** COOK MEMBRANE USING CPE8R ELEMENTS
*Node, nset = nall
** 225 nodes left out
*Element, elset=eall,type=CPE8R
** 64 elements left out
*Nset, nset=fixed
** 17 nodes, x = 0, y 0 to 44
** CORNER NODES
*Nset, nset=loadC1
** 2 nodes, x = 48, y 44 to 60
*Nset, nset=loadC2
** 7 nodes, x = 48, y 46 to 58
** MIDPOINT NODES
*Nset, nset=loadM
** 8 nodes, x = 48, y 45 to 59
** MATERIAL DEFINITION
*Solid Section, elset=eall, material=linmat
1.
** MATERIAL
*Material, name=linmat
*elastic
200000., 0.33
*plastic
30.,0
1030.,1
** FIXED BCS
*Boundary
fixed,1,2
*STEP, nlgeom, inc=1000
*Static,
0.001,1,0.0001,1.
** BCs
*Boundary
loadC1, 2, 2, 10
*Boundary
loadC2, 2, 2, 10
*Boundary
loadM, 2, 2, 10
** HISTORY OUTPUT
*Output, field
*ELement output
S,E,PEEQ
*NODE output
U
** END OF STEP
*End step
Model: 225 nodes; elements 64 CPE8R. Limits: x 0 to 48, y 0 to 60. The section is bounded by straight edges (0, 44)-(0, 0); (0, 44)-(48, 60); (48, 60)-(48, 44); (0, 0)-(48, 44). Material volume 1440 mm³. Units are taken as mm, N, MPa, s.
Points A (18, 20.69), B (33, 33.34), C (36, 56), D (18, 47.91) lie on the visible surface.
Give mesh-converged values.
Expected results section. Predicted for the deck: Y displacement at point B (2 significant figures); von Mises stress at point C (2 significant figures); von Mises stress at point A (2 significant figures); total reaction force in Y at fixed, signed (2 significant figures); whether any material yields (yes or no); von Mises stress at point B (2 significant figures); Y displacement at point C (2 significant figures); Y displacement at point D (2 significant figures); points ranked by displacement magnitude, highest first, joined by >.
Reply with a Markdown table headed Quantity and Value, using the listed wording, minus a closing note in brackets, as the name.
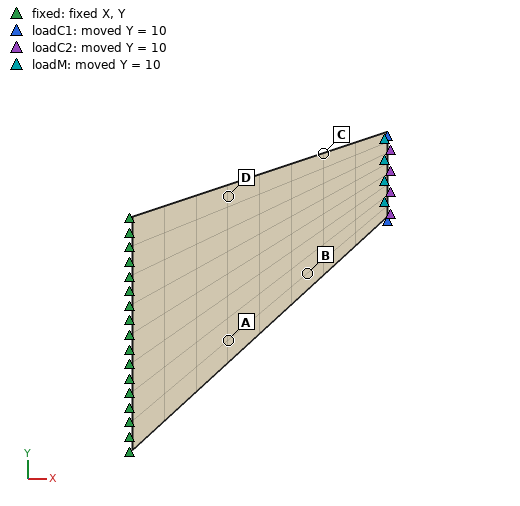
| Quantity | Value |
|---|---|
| Y displacement at point B | 4.7 mm |
| von Mises stress at point C | 80 MPa |
| von Mises stress at point A | 120 MPa |
| total reaction force in Y at fixed, signed | -950 N |
| whether any material yields | yes |
| von Mises stress at point B | 140 MPa |
| Y displacement at point C | 5.3 mm |
| Y displacement at point D | 1.5 mm |
| points ranked by displacement magnitude, highest first, joined by > | C > B > D > A |
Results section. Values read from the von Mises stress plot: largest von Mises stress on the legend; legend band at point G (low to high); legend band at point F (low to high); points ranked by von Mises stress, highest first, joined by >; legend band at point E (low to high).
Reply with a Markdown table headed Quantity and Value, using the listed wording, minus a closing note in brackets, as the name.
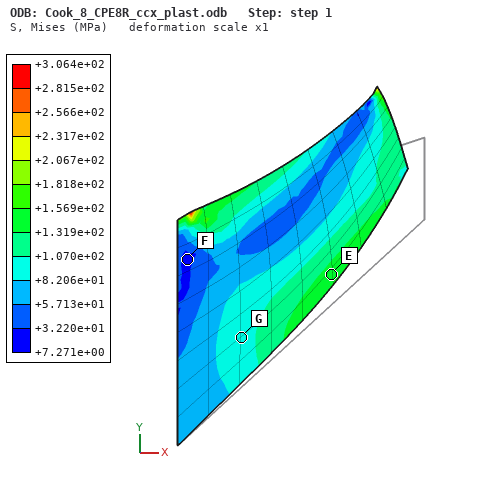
| Quantity | Value |
|---|---|
| largest von Mises stress on the legend | +3.064e+02 MPa |
| legend band at point G | +8.206e+01 to +1.070e+02 MPa |
| legend band at point F | +7.271e+00 to +3.220e+01 MPa |
| points ranked by von Mises stress, highest first, joined by > | E > G > F |
| legend band at point E | +1.319e+02 to +1.569e+02 MPa |
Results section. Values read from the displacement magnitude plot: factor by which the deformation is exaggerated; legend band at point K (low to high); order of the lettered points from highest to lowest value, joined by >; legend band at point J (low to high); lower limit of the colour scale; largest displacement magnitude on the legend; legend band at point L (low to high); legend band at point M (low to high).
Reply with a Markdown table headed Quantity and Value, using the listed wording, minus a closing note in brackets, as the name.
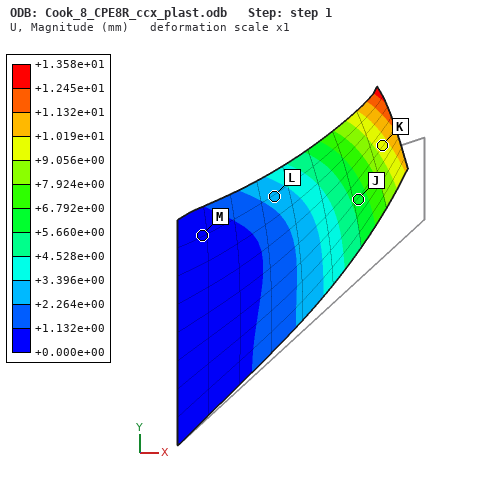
| Quantity | Value |
|---|---|
| factor by which the deformation is exaggerated | 1 |
| legend band at point K | +9.056e+00 to +1.019e+01 mm |
| order of the lettered points from highest to lowest value, joined by > | K > J > L > M |
| legend band at point J | +5.660e+00 to +6.792e+00 mm |
| lower limit of the colour scale | +0.000e+00 mm |
| largest displacement magnitude on the legend | +1.358e+01 mm |
| legend band at point L | +2.264e+00 to +3.396e+00 mm |
| legend band at point M | +0.000e+00 to +1.132e+00 mm |
